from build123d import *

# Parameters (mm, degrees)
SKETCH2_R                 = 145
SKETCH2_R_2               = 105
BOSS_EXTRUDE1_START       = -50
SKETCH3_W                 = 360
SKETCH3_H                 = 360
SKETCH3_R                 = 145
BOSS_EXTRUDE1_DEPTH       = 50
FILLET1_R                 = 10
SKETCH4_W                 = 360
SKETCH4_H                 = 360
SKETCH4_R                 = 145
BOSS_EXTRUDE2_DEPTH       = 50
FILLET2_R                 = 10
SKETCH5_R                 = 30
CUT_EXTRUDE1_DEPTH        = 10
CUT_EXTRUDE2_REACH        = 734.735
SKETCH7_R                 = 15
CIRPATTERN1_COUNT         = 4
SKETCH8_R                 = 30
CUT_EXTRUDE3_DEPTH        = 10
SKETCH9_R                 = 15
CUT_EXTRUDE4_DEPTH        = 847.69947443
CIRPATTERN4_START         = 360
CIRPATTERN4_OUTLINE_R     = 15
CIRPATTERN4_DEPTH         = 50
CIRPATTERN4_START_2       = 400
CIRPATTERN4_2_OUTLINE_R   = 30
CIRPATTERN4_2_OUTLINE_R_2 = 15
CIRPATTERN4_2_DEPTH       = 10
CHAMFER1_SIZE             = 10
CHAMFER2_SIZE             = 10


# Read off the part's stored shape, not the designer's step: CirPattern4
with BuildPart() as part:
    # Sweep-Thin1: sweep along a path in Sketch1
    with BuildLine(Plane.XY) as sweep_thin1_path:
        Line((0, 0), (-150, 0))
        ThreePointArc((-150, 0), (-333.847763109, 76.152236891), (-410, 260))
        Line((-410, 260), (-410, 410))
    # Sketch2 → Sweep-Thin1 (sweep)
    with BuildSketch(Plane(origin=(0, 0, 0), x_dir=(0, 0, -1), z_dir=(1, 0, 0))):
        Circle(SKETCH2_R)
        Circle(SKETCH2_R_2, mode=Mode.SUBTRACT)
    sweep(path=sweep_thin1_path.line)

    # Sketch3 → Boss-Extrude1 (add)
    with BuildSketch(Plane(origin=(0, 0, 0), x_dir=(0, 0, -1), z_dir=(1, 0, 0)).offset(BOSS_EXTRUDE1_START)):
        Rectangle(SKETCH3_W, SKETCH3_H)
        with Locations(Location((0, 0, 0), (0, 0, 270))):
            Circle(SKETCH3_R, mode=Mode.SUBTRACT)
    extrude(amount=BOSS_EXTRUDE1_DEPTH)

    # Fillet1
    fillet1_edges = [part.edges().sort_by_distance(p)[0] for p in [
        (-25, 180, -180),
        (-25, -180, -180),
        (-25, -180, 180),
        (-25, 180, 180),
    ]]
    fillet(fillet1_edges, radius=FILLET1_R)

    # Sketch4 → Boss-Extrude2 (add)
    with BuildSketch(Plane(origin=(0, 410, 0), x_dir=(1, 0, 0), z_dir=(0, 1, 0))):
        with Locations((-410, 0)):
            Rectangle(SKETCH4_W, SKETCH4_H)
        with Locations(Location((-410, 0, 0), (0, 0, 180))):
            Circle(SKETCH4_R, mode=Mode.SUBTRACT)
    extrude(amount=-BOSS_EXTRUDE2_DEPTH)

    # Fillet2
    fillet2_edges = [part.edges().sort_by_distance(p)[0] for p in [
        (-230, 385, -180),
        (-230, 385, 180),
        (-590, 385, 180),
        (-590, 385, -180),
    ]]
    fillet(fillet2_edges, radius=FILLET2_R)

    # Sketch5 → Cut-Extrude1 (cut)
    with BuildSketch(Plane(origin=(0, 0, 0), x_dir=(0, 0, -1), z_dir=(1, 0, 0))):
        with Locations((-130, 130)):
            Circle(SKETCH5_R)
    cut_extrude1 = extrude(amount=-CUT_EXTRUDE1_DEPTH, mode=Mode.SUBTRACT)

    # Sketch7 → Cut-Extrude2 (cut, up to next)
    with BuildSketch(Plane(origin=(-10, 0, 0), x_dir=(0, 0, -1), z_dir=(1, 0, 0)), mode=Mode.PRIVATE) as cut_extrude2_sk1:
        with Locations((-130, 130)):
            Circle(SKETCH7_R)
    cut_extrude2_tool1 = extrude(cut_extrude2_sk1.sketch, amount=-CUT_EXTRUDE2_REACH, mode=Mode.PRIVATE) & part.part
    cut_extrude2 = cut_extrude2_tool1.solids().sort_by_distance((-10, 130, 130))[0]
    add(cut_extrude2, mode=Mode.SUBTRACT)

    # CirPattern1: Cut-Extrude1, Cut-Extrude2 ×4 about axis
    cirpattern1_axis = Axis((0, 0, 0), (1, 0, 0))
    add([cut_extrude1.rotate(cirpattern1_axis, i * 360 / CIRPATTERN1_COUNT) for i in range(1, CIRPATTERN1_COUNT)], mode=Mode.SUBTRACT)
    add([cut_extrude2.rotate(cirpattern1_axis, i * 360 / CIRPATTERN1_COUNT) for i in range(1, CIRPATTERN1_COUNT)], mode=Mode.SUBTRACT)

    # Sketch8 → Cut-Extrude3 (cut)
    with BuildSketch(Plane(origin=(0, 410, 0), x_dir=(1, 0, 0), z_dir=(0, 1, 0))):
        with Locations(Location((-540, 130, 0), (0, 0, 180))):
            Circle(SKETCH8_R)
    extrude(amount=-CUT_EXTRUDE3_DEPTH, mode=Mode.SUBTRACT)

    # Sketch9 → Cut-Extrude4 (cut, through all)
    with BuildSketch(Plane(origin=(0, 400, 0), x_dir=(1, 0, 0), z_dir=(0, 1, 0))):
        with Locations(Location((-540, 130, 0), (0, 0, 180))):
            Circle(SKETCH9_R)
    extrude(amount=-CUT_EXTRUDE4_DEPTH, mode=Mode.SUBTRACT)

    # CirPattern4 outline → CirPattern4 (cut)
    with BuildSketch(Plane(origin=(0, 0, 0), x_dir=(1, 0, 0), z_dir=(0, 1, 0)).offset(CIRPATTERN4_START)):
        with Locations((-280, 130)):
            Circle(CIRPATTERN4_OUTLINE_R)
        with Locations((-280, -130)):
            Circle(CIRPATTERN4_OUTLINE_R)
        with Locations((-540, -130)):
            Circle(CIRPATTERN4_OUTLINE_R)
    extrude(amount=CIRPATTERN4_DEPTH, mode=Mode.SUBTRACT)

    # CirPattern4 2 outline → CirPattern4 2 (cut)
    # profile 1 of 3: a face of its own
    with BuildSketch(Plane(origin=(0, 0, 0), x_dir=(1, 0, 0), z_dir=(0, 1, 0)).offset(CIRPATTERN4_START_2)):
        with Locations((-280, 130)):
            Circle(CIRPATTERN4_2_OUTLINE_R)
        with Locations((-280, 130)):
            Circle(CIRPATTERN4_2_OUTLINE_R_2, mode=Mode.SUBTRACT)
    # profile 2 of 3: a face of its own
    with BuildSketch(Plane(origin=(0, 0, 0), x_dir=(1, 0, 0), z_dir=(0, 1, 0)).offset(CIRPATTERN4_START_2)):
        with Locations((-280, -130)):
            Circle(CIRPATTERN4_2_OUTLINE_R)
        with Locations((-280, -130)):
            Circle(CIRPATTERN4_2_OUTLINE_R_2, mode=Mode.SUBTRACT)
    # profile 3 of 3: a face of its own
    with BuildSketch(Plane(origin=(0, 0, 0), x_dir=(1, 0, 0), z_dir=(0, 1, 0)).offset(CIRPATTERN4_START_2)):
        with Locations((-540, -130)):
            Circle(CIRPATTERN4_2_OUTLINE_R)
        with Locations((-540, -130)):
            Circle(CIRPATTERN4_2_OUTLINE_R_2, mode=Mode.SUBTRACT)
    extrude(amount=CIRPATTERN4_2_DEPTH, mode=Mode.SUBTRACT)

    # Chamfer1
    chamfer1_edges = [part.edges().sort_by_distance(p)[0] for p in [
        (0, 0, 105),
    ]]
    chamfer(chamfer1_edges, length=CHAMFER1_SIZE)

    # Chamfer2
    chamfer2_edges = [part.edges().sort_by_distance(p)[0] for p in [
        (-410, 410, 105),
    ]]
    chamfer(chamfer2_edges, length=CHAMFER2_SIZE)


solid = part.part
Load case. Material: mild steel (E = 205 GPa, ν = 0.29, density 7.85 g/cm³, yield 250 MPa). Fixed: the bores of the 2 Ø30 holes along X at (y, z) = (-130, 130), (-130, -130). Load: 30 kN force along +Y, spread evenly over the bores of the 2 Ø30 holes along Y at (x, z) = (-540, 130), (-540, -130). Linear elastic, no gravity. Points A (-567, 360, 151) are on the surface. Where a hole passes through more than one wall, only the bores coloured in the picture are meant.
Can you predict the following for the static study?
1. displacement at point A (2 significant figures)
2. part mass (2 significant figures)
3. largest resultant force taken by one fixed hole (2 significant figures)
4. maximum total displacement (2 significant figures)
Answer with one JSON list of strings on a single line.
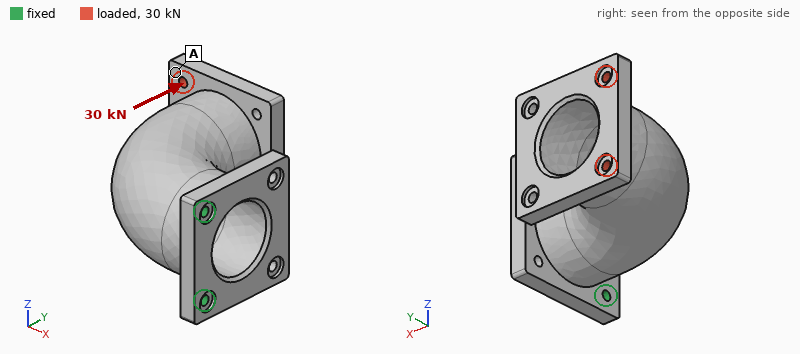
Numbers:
["1.5 mm", "220 kg", "15 kN", "1.6 mm"]
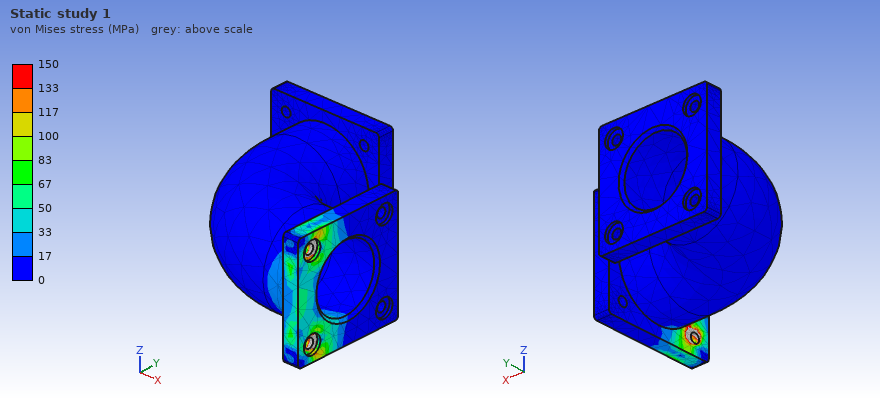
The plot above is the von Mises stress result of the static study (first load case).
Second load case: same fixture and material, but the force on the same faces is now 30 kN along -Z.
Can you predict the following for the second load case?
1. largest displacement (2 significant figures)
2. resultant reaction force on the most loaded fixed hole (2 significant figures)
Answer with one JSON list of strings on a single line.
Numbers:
["0.25 mm", "85 kN"]
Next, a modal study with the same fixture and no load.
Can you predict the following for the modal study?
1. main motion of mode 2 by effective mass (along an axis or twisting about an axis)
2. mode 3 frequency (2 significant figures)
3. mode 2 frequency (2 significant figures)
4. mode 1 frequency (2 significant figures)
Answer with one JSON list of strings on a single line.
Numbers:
["along Z", "550 Hz", "220 Hz", "69 Hz"]
